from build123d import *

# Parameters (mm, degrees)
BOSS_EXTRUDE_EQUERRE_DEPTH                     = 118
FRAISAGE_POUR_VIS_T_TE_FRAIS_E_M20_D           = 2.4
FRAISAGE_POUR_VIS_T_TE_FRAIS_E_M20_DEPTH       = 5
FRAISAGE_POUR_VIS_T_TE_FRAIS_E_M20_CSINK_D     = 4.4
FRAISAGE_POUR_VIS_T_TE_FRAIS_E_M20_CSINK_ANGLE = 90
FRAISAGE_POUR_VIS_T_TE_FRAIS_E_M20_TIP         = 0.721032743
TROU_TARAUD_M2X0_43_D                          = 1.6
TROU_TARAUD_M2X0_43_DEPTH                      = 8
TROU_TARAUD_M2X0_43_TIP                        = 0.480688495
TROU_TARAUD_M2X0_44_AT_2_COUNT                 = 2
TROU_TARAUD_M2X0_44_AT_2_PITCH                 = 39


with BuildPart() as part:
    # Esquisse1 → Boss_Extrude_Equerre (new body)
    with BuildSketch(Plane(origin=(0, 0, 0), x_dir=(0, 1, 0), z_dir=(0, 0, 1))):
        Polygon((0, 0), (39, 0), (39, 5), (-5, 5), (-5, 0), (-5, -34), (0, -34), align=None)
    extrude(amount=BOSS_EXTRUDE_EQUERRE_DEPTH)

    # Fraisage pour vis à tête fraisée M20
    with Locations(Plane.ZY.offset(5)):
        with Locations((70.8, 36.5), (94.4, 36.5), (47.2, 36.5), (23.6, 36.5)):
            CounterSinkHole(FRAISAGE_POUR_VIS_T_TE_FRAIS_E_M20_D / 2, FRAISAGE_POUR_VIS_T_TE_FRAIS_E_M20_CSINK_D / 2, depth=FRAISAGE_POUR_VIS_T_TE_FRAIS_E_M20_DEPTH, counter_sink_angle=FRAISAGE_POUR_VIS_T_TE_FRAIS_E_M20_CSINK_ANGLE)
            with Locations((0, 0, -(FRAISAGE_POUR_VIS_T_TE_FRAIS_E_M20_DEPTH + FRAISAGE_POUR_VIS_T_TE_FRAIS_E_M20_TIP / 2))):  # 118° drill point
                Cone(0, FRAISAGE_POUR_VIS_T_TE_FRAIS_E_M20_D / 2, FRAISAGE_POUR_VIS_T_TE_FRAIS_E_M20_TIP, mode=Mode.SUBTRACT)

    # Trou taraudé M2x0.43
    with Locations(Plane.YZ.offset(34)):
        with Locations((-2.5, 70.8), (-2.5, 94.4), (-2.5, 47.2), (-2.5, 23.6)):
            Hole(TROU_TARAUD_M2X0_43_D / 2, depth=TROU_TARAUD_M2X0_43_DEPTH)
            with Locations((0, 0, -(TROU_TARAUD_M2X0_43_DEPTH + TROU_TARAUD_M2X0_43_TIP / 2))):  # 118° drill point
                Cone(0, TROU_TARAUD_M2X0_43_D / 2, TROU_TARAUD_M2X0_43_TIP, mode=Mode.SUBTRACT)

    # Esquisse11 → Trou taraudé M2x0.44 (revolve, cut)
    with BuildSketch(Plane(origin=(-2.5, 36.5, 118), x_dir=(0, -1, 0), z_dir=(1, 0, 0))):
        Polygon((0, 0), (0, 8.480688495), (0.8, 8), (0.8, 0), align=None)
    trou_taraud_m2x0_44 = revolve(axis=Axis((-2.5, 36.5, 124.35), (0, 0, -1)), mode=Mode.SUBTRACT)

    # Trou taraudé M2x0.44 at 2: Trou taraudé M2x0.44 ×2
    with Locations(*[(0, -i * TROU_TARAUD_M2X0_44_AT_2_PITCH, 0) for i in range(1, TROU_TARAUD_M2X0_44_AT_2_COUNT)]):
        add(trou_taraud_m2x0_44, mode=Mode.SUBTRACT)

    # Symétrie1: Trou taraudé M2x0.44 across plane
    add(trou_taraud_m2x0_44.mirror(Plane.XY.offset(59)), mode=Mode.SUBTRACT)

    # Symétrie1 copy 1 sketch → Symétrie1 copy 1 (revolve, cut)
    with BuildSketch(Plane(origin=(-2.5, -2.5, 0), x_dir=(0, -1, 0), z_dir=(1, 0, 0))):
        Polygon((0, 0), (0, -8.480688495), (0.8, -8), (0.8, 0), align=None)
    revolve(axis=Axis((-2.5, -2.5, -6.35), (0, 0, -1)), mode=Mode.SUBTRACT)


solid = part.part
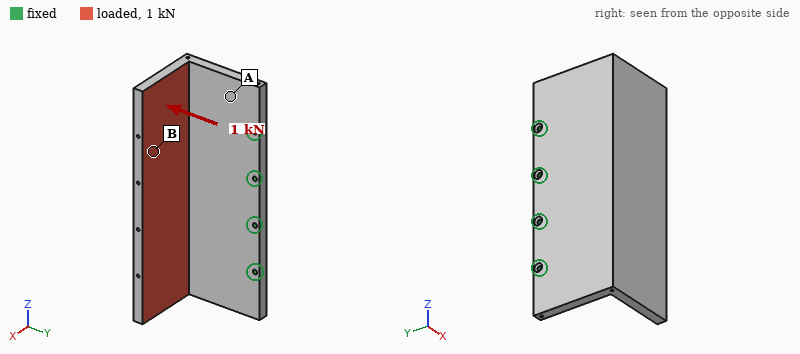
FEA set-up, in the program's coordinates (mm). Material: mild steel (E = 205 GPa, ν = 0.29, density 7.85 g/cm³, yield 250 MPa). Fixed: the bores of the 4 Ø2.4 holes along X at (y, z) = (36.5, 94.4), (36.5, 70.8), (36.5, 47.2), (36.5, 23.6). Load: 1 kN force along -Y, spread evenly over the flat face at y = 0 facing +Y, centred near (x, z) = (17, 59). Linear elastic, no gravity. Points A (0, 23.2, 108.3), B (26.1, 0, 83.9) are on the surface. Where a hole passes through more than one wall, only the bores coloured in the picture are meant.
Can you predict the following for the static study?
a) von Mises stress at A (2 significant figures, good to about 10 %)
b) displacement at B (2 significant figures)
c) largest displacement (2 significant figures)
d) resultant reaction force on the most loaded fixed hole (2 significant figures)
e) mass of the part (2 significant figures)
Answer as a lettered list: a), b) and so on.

a) 33 MPa
b) 0.14 mm
c) 0.19 mm
d) 280 N
e) 360 g
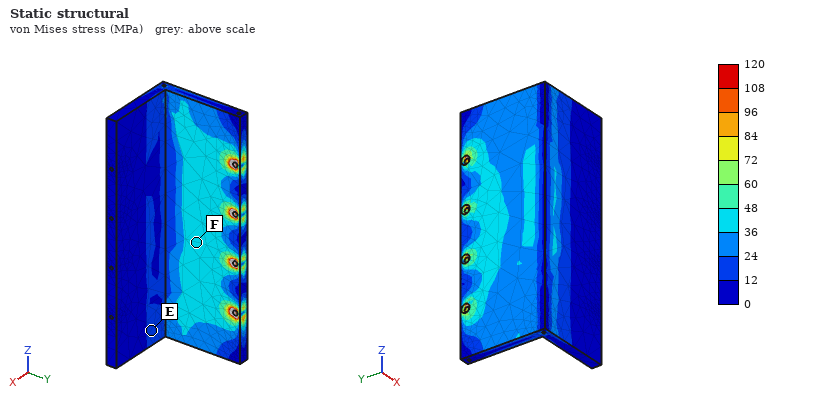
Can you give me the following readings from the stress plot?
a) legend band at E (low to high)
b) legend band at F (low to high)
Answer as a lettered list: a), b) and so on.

a) 12 to 24 MPa
b) 36 to 48 MPa
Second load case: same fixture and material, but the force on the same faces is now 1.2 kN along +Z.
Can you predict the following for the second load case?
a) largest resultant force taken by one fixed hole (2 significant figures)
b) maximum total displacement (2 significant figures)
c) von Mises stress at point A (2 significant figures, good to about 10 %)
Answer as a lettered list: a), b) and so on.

a) 680 N
b) 92 µm
c) 12 MPa
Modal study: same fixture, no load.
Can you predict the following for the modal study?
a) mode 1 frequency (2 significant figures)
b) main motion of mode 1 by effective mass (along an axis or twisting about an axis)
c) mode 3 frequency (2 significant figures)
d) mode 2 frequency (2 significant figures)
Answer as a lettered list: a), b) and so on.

a) 770 Hz
b) along X
c) 2500 Hz
d) 1200 Hz
